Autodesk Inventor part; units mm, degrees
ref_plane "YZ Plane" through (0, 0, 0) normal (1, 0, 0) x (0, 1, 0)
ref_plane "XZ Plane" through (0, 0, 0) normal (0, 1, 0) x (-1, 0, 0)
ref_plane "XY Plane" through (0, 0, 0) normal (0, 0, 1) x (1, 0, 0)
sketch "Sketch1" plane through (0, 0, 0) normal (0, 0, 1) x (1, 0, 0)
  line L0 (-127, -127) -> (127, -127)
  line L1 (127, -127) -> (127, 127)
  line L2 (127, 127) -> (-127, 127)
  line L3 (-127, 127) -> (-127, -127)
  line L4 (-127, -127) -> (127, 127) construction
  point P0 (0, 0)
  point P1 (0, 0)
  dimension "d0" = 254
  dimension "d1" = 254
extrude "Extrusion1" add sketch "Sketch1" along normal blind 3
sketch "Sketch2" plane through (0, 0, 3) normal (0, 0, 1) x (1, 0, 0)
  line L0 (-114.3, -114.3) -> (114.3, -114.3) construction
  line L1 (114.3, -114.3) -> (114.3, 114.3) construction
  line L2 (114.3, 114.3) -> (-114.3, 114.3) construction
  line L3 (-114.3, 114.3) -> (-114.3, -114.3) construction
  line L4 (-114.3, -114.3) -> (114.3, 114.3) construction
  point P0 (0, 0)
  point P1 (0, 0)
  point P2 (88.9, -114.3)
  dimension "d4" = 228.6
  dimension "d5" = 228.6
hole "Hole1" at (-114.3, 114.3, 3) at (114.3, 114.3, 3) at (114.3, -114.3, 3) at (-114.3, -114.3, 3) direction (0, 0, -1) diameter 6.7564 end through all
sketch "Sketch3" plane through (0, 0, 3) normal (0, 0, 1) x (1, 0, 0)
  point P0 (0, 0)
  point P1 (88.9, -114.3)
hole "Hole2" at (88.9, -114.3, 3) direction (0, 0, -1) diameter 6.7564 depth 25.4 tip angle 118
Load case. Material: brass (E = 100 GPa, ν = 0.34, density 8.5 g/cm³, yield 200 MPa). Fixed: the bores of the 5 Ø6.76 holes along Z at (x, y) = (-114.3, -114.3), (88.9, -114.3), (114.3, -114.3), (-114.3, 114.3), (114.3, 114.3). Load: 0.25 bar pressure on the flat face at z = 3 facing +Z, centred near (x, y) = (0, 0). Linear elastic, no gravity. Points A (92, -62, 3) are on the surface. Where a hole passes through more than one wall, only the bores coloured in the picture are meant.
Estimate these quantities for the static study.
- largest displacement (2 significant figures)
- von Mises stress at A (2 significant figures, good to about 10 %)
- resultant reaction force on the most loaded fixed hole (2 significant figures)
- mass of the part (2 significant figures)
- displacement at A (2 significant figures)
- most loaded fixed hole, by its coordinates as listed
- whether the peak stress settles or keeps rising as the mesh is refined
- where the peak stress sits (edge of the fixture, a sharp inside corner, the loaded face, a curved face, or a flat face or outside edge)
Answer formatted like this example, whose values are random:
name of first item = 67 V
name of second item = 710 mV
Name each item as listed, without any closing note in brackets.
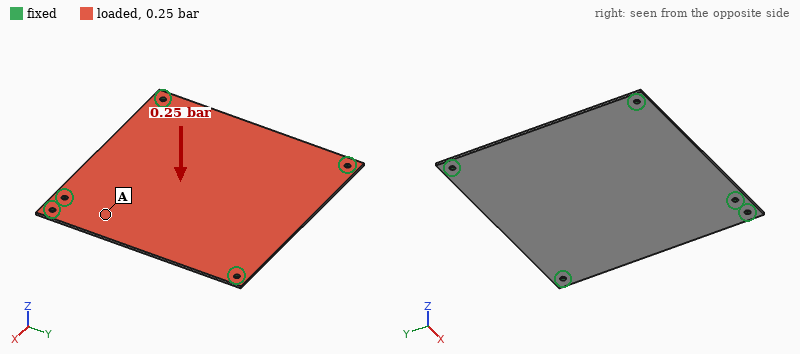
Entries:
largest displacement = 2.0 mm
von Mises stress at A = 21 MPa
resultant reaction force on the most loaded fixed hole = 510 N
mass of the part = 1.6 kg
displacement at A = 0.65 mm
most loaded fixed hole, by its coordinates as listed = (88.9, -114.3)
whether the peak stress settles or keeps rising as the mesh is refined = keeps rising
where the peak stress sits = edge of the fixture
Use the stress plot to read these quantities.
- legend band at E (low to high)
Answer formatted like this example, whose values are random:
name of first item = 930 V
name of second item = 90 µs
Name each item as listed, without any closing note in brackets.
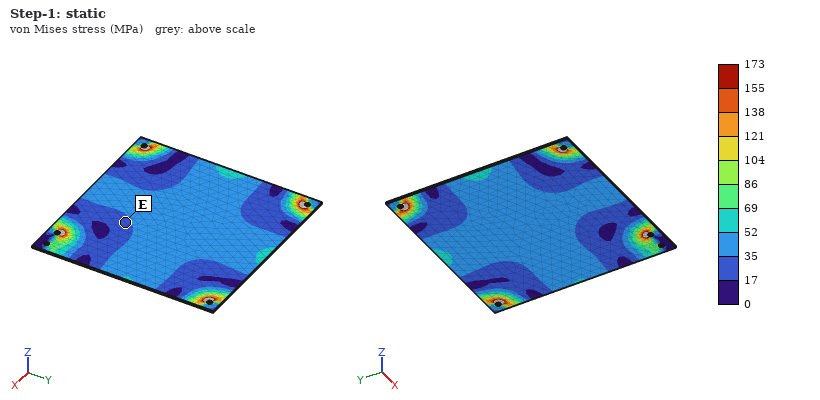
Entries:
legend band at E = 17 to 35 MPa
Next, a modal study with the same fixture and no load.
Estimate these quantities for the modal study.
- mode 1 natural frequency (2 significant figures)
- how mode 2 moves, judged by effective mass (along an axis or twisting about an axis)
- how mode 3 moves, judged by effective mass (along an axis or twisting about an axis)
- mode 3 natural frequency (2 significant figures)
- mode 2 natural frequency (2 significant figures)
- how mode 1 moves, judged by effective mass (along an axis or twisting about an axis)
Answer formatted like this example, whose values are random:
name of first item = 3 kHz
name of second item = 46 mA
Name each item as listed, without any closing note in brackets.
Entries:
mode 1 natural frequency = 130 Hz
how mode 2 moves, judged by effective mass = twisting about Y
how mode 3 moves, judged by effective mass = twisting about X
mode 3 natural frequency = 240 Hz
mode 2 natural frequency = 220 Hz
how mode 1 moves, judged by effective mass = along Z
